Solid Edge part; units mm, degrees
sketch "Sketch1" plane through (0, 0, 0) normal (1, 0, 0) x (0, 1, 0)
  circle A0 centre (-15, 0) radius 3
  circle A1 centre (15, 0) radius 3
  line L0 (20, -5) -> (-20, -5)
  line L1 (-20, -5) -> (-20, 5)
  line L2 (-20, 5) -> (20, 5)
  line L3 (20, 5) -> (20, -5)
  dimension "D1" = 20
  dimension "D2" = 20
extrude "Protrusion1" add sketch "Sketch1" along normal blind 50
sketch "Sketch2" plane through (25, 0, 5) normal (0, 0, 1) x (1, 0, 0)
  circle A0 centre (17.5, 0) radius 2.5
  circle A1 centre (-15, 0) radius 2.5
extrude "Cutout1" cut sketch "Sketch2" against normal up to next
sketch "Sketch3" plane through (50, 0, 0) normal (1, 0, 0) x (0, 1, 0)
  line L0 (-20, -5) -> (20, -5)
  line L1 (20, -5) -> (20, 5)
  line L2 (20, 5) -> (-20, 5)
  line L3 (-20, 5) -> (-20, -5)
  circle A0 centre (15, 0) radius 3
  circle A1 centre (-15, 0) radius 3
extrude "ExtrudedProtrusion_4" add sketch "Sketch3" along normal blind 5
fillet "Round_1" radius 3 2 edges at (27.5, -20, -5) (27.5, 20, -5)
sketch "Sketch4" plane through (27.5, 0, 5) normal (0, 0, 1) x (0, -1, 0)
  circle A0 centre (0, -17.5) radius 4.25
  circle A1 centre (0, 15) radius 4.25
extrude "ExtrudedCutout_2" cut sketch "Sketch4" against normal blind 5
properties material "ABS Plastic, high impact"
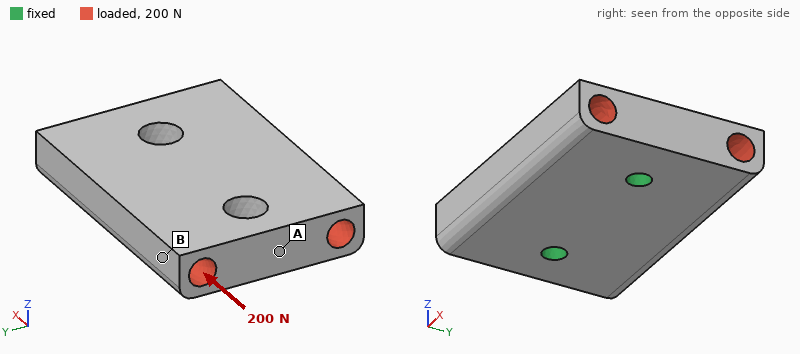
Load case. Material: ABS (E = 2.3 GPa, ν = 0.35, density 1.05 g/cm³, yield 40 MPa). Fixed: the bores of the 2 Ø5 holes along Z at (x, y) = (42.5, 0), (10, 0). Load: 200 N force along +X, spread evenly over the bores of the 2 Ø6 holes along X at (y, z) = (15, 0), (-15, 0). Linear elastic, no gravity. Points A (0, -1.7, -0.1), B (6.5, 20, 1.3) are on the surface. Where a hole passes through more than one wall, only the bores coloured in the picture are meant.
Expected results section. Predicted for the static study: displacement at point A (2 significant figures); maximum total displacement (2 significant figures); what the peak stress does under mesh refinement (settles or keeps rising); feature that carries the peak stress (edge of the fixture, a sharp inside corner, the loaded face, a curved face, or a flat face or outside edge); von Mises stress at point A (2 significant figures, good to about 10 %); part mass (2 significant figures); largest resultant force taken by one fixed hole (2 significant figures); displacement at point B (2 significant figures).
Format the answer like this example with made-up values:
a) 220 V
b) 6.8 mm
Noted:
a) 3.4 µm
b) 9.2 µm
c) keeps rising
d) edge of the fixture
e) 0.67 MPa
f) 19 g
g) 100 N
h) 8.1 µm
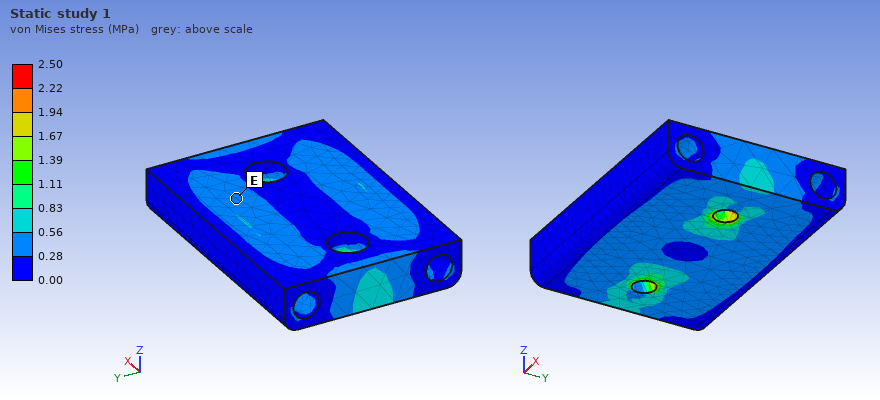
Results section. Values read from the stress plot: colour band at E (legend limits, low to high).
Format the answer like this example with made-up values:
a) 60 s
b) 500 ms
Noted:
a) 0.28 to 0.56 MPa
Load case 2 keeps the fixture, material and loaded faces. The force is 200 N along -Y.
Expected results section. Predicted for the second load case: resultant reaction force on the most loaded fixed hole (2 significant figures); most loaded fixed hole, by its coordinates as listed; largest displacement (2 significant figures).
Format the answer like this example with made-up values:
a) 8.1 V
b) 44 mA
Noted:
a) 110 N
b) (42.5, 0)
c) 23 µm
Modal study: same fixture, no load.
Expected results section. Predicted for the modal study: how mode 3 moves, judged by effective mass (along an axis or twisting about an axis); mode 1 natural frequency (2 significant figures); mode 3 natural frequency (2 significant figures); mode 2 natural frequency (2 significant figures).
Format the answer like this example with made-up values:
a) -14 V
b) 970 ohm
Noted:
a) along Z
b) 2300 Hz
c) 4700 Hz
d) 4500 Hz
